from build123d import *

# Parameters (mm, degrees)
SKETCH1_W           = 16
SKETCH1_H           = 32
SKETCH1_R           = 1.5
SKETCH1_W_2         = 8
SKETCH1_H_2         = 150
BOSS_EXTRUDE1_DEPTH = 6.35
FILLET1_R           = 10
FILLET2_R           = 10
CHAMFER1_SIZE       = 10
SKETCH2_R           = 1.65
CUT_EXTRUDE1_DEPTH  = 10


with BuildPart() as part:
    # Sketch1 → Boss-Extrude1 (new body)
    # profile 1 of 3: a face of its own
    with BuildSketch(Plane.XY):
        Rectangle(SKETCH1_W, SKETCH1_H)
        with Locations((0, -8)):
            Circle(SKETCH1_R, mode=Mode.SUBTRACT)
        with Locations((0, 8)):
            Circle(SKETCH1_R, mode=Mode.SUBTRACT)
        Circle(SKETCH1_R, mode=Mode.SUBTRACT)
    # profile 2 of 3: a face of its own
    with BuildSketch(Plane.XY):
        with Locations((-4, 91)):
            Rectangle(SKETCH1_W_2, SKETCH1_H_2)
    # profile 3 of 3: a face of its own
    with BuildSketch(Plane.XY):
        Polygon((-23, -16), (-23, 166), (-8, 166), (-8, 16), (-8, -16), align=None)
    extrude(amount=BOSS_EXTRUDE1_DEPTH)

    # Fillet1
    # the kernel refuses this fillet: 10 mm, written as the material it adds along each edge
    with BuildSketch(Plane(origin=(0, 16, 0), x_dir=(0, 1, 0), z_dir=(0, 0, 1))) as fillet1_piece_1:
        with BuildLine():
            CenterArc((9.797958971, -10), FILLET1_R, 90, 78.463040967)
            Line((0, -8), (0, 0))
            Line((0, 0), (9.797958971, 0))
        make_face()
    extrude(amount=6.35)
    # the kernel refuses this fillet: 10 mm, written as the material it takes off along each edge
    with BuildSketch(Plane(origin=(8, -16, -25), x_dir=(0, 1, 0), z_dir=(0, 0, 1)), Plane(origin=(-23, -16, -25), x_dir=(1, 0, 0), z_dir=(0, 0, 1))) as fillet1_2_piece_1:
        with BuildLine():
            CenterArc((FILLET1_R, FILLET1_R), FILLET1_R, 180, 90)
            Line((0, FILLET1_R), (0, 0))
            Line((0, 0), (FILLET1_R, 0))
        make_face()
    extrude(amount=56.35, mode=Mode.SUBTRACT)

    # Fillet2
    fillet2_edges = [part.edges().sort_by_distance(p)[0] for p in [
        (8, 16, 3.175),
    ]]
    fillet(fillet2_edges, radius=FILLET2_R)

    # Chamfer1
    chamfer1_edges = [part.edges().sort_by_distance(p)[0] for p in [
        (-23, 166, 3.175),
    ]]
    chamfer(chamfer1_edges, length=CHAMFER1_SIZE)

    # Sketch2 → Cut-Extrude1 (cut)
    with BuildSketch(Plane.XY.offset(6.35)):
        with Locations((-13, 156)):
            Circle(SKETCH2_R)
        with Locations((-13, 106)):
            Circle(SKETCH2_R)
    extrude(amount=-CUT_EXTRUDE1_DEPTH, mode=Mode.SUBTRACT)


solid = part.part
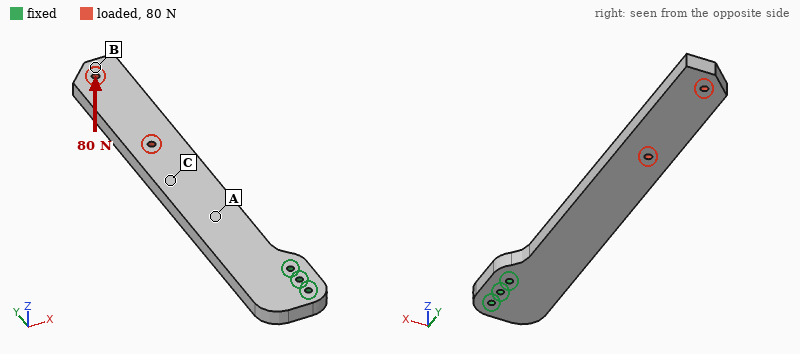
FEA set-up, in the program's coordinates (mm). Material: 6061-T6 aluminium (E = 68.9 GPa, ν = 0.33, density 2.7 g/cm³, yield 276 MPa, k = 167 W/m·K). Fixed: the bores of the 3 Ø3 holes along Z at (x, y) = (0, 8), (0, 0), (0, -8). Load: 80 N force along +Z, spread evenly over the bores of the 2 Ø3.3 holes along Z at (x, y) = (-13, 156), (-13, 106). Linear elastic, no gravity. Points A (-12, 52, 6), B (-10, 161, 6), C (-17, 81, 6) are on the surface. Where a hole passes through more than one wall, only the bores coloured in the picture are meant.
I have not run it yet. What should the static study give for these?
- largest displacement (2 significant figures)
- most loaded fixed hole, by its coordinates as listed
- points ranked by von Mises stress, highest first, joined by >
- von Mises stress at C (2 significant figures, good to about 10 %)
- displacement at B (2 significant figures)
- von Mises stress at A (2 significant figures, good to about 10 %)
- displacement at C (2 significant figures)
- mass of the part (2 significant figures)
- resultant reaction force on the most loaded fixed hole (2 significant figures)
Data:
2.2 mm
(0, 8)
A > C > B
26 MPa
2.1 mm
41 MPa
0.66 mm
74 g
510 N
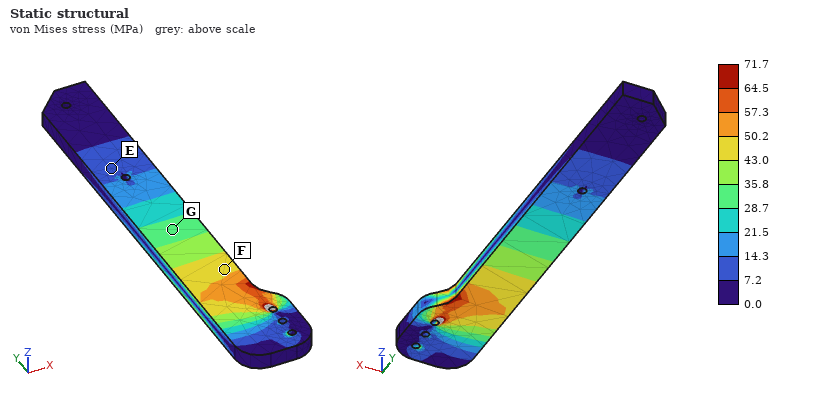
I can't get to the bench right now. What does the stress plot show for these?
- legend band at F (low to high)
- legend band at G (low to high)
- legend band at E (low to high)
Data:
43.0 to 50.2 MPa
28.7 to 35.8 MPa
7.2 to 14.3 MPa
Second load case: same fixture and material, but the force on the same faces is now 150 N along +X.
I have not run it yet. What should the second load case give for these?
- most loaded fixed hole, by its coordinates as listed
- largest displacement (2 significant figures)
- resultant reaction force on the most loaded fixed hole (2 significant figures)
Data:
(0, 8)
0.34 mm
1.2 kN
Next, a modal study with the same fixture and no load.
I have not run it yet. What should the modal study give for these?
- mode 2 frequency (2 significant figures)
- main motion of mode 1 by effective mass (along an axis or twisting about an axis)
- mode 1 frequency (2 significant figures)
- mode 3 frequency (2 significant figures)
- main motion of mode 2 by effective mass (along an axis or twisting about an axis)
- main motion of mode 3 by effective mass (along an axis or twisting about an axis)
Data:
720 Hz
along Z
210 Hz
1300 Hz
along X
along Z
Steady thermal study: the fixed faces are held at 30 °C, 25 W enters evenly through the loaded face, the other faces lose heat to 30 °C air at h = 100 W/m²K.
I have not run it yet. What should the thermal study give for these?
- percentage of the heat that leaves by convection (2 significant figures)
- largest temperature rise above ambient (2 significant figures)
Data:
80 %
43 K
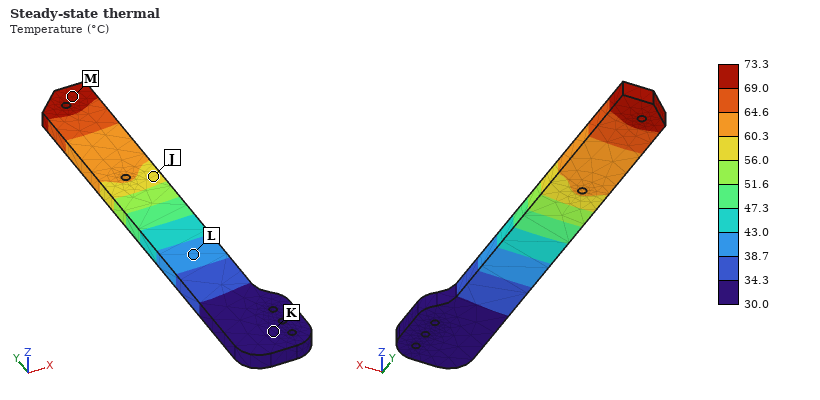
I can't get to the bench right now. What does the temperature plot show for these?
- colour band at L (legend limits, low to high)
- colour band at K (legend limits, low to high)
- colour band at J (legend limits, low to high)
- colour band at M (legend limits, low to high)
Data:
38.7 to 43.0 °C
30.0 to 34.3 °C
56.0 to 60.3 °C
69.0 to 73.3 °C
